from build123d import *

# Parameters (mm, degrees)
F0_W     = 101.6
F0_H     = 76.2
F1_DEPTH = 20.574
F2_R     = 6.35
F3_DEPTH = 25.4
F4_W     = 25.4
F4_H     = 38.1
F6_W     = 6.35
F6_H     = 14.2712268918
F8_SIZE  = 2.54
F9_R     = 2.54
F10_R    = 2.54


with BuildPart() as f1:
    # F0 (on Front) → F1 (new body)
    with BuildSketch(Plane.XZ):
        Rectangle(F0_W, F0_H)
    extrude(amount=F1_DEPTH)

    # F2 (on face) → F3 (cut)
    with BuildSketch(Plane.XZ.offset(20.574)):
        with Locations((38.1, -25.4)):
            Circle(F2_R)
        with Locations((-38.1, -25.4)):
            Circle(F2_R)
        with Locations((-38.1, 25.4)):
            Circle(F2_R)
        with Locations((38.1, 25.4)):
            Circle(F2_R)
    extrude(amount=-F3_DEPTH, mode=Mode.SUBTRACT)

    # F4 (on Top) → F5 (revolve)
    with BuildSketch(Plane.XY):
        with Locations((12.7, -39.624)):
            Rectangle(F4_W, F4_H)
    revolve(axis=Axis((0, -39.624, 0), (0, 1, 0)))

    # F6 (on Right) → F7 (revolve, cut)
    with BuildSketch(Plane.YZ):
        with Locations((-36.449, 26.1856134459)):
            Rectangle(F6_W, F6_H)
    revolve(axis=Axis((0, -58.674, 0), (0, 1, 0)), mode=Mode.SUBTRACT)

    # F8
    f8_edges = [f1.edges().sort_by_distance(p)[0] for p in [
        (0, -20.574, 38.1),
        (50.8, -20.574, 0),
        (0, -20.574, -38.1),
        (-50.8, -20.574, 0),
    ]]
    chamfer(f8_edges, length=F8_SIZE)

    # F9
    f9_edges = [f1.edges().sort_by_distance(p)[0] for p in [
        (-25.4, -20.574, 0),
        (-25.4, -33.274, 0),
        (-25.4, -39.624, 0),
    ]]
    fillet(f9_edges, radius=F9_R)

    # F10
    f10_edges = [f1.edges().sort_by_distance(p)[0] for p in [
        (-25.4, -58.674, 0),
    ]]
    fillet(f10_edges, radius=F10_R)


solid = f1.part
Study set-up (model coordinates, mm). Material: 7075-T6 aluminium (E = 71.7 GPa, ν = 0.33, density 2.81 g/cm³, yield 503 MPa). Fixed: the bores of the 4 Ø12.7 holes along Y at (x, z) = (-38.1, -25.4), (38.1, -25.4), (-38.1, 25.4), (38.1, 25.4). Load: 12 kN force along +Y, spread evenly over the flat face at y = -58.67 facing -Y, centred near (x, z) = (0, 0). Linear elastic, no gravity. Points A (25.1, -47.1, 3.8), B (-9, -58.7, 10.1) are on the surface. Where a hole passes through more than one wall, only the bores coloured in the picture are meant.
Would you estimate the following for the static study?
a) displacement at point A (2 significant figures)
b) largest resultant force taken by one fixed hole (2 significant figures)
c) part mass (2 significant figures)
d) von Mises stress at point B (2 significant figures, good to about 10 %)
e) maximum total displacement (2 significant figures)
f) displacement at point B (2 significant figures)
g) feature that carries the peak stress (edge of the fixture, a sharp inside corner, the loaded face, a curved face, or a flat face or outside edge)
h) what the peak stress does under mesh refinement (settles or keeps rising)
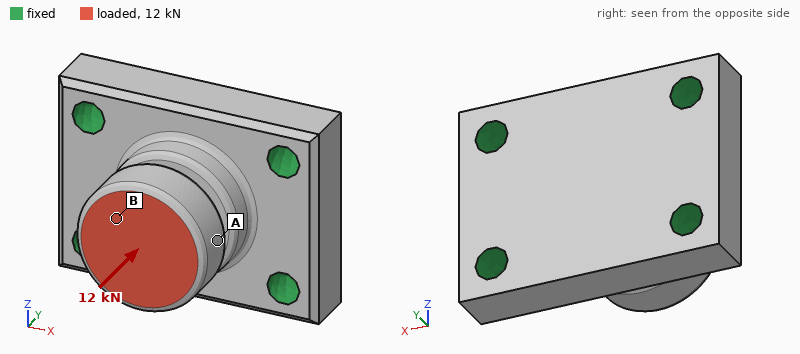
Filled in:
10 µm
3.1 kN
620 g
7.5 MPa
11 µm
11 µm
edge of the fixture
keeps rising
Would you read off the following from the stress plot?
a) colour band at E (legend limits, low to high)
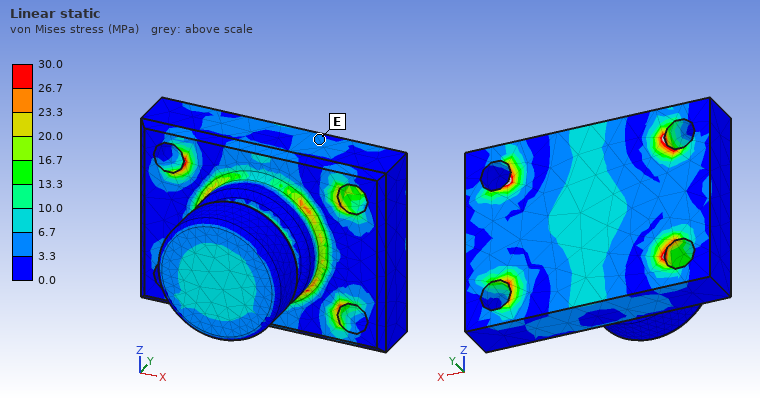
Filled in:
3.3 to 6.7 MPa
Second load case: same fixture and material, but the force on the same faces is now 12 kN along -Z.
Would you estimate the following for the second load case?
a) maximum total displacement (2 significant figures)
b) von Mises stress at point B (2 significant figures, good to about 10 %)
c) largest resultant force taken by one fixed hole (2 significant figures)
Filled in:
69 µm
15 MPa
6.6 kN
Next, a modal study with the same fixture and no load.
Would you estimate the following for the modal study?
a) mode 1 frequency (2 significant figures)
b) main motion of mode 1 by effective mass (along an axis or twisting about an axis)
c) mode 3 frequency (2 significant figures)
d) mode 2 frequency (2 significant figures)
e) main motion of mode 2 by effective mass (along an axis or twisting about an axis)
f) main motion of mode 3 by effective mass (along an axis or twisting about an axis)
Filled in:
7500 Hz
along Z
11 kHz
9000 Hz
along X
along Y
